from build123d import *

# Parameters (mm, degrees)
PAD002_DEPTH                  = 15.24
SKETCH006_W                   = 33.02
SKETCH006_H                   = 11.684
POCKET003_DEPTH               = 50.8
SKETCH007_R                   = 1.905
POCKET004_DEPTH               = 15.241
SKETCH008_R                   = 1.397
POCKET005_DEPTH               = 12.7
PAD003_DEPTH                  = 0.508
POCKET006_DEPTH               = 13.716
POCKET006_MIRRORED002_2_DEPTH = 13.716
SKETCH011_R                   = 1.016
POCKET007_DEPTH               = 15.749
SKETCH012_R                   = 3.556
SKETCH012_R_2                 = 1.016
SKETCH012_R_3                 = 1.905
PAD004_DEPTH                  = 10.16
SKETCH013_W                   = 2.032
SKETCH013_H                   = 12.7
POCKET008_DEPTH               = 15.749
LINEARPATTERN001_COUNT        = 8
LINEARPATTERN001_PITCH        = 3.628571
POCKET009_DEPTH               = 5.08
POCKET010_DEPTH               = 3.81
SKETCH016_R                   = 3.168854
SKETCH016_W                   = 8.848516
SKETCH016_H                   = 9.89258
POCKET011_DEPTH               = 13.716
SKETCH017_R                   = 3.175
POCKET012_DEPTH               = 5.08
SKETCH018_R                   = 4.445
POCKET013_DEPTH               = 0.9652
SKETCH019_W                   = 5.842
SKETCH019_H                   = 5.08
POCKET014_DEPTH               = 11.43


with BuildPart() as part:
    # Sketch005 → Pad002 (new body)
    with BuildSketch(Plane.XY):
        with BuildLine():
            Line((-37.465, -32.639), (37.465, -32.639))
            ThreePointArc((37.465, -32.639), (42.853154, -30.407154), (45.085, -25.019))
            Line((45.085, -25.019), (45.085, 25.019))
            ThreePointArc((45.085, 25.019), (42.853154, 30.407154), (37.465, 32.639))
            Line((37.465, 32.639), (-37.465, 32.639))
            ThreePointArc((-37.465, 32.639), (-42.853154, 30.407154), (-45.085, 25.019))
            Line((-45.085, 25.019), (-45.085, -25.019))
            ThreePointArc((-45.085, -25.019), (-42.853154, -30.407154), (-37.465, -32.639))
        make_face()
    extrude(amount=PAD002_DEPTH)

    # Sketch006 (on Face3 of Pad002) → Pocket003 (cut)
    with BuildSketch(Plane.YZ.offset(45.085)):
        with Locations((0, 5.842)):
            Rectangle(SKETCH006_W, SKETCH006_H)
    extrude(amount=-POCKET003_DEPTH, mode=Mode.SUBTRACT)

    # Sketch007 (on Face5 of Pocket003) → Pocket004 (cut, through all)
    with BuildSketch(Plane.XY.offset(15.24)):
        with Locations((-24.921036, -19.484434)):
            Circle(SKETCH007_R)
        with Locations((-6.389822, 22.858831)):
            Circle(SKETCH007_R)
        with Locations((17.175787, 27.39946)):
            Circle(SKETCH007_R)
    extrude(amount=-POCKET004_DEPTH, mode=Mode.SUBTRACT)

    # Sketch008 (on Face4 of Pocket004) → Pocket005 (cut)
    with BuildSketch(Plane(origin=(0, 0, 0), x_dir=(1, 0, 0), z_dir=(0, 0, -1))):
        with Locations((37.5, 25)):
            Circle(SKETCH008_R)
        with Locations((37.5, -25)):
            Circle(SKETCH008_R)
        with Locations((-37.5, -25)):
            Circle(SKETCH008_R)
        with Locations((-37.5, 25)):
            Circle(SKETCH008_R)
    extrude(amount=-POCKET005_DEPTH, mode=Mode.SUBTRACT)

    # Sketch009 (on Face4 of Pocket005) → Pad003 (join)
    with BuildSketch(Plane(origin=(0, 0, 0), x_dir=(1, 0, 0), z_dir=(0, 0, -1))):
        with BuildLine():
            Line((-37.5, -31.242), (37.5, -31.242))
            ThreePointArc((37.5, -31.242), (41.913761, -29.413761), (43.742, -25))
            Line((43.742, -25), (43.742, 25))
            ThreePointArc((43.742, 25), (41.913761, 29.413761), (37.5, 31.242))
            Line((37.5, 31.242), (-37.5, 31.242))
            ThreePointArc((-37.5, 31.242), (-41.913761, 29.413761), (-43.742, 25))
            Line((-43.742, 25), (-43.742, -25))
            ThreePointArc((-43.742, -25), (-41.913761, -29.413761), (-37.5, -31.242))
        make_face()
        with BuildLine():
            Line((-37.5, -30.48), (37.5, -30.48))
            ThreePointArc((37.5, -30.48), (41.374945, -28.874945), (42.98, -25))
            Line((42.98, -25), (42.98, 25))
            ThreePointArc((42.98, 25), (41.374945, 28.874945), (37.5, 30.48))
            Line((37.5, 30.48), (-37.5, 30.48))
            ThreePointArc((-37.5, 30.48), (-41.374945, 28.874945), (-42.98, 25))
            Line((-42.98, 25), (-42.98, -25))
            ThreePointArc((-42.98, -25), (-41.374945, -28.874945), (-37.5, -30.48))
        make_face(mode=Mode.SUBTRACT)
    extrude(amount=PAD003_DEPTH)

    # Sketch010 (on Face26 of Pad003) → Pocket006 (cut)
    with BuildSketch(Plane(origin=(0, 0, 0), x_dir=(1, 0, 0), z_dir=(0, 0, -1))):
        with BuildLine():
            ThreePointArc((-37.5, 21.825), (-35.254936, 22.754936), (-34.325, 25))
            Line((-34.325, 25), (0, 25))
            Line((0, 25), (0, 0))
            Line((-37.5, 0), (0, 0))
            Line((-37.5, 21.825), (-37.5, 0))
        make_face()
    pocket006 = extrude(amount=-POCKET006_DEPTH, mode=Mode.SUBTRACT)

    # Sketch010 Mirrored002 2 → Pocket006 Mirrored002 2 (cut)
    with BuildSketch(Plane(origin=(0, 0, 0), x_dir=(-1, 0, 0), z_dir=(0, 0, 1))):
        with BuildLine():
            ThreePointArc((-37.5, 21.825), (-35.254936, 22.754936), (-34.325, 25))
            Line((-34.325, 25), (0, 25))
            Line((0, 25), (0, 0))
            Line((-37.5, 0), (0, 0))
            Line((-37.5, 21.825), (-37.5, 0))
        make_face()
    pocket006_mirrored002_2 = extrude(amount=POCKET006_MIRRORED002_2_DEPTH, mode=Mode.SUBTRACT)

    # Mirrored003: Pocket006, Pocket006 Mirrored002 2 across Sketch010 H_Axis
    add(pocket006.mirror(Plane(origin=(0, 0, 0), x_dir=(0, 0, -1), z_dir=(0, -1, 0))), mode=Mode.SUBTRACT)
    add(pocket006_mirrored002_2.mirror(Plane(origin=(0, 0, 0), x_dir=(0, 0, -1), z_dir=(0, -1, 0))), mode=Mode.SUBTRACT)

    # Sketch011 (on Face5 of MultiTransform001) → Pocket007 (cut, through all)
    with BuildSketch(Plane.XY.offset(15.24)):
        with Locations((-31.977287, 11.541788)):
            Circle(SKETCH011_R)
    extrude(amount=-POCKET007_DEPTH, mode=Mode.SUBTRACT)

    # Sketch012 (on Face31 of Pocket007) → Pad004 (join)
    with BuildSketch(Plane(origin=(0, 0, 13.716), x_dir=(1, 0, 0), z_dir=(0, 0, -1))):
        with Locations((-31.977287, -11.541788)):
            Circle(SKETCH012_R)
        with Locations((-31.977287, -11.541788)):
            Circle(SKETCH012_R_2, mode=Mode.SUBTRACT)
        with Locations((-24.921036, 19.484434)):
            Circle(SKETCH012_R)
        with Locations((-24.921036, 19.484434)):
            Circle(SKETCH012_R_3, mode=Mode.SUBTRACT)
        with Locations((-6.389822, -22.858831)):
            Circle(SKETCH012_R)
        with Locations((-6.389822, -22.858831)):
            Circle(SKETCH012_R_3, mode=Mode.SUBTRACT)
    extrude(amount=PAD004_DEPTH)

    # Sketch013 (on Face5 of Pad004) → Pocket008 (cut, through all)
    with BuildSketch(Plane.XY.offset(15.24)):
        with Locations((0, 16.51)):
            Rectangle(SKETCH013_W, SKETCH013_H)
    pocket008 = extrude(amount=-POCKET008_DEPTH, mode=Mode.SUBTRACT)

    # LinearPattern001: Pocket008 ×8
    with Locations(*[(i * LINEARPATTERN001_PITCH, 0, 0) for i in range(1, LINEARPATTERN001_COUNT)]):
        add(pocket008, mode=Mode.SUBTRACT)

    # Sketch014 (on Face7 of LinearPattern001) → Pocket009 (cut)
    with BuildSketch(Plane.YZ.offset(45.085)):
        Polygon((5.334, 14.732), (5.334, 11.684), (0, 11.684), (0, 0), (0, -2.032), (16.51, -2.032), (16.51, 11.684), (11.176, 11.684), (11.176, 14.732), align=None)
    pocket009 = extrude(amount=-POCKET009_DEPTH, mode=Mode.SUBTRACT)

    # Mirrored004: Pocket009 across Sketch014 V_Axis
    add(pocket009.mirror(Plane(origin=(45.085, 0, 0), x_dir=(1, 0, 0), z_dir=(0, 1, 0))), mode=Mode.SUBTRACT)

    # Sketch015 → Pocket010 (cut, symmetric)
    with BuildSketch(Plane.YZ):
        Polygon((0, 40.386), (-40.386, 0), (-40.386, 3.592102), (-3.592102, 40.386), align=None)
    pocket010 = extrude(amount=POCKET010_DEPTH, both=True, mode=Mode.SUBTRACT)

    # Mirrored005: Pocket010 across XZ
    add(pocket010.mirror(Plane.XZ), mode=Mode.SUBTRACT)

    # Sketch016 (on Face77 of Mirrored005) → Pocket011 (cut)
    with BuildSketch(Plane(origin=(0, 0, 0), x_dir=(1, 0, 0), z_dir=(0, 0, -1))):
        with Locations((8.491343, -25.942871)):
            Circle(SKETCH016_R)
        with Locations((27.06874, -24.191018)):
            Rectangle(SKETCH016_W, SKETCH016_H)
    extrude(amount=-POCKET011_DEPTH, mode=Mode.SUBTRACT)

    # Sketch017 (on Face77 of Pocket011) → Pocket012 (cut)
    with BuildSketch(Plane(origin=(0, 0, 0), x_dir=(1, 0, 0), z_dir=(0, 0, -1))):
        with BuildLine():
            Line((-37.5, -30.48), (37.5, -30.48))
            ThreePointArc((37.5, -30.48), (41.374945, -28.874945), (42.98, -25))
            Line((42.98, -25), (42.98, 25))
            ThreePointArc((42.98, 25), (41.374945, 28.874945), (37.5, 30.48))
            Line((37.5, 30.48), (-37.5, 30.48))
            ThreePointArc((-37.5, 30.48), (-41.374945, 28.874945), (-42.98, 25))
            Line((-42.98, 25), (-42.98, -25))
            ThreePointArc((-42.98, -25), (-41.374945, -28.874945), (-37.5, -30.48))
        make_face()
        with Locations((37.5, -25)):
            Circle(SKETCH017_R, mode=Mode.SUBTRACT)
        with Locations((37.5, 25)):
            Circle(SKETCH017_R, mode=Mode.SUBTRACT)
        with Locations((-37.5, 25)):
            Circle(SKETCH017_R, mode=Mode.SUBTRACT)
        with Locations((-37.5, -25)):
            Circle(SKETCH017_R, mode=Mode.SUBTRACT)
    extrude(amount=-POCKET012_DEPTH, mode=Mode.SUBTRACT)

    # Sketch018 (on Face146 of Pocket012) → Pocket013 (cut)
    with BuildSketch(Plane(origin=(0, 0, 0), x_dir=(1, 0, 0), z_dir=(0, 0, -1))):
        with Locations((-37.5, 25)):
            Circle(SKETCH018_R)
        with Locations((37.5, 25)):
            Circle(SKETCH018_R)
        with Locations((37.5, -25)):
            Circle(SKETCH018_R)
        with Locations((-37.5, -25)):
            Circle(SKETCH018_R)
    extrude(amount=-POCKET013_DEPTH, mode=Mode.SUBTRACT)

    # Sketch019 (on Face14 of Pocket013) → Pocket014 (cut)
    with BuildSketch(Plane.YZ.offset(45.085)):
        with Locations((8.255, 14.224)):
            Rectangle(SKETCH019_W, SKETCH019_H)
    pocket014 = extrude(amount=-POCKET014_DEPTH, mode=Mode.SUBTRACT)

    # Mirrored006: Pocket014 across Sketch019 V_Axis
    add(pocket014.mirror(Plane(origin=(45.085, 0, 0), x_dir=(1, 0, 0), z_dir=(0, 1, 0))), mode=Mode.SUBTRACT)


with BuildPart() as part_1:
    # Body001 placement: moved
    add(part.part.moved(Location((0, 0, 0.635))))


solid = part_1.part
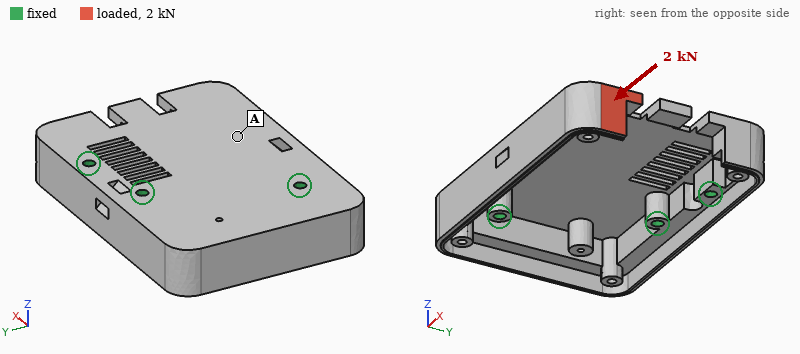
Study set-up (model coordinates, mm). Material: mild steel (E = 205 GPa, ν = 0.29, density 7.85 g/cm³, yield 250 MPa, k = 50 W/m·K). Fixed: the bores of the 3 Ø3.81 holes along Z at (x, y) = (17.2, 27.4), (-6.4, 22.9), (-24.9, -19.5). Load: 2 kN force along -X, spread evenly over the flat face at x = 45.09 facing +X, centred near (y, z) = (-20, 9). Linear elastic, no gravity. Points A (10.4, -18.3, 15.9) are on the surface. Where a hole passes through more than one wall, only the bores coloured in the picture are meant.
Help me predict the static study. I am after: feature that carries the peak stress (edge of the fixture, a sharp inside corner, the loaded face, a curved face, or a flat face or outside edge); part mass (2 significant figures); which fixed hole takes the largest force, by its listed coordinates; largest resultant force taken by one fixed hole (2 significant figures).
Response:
a flat face or outside edge
220 g
(-24.9, -19.5)
1.9 kN
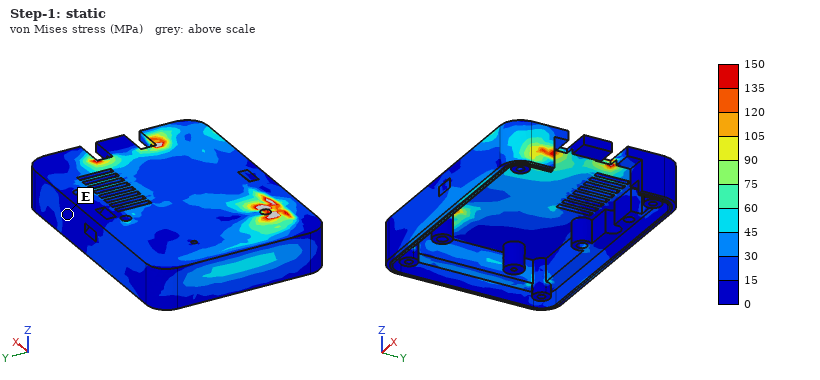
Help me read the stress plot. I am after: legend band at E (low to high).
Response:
0 to 15 MPa
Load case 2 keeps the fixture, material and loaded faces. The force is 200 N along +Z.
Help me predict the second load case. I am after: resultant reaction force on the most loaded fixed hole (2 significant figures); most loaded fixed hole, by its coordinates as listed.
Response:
420 N
(-6.4, 22.9)
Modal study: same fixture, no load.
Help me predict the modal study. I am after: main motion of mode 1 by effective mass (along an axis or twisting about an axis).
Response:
along Z
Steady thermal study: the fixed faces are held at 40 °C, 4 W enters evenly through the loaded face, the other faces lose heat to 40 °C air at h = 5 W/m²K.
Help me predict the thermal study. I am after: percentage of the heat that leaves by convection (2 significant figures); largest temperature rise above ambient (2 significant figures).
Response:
21 %
43 K
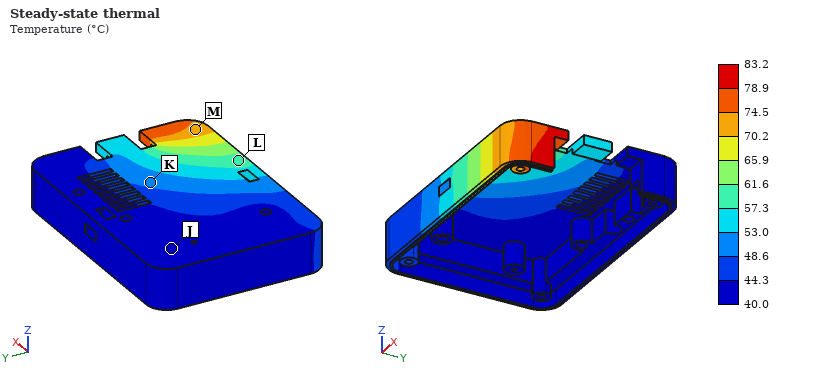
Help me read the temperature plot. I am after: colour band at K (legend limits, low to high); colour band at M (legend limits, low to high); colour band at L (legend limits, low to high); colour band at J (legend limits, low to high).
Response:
48.6 to 53.0 °C
70.2 to 74.5 °C
57.3 to 61.6 °C
40.0 to 44.3 °C
